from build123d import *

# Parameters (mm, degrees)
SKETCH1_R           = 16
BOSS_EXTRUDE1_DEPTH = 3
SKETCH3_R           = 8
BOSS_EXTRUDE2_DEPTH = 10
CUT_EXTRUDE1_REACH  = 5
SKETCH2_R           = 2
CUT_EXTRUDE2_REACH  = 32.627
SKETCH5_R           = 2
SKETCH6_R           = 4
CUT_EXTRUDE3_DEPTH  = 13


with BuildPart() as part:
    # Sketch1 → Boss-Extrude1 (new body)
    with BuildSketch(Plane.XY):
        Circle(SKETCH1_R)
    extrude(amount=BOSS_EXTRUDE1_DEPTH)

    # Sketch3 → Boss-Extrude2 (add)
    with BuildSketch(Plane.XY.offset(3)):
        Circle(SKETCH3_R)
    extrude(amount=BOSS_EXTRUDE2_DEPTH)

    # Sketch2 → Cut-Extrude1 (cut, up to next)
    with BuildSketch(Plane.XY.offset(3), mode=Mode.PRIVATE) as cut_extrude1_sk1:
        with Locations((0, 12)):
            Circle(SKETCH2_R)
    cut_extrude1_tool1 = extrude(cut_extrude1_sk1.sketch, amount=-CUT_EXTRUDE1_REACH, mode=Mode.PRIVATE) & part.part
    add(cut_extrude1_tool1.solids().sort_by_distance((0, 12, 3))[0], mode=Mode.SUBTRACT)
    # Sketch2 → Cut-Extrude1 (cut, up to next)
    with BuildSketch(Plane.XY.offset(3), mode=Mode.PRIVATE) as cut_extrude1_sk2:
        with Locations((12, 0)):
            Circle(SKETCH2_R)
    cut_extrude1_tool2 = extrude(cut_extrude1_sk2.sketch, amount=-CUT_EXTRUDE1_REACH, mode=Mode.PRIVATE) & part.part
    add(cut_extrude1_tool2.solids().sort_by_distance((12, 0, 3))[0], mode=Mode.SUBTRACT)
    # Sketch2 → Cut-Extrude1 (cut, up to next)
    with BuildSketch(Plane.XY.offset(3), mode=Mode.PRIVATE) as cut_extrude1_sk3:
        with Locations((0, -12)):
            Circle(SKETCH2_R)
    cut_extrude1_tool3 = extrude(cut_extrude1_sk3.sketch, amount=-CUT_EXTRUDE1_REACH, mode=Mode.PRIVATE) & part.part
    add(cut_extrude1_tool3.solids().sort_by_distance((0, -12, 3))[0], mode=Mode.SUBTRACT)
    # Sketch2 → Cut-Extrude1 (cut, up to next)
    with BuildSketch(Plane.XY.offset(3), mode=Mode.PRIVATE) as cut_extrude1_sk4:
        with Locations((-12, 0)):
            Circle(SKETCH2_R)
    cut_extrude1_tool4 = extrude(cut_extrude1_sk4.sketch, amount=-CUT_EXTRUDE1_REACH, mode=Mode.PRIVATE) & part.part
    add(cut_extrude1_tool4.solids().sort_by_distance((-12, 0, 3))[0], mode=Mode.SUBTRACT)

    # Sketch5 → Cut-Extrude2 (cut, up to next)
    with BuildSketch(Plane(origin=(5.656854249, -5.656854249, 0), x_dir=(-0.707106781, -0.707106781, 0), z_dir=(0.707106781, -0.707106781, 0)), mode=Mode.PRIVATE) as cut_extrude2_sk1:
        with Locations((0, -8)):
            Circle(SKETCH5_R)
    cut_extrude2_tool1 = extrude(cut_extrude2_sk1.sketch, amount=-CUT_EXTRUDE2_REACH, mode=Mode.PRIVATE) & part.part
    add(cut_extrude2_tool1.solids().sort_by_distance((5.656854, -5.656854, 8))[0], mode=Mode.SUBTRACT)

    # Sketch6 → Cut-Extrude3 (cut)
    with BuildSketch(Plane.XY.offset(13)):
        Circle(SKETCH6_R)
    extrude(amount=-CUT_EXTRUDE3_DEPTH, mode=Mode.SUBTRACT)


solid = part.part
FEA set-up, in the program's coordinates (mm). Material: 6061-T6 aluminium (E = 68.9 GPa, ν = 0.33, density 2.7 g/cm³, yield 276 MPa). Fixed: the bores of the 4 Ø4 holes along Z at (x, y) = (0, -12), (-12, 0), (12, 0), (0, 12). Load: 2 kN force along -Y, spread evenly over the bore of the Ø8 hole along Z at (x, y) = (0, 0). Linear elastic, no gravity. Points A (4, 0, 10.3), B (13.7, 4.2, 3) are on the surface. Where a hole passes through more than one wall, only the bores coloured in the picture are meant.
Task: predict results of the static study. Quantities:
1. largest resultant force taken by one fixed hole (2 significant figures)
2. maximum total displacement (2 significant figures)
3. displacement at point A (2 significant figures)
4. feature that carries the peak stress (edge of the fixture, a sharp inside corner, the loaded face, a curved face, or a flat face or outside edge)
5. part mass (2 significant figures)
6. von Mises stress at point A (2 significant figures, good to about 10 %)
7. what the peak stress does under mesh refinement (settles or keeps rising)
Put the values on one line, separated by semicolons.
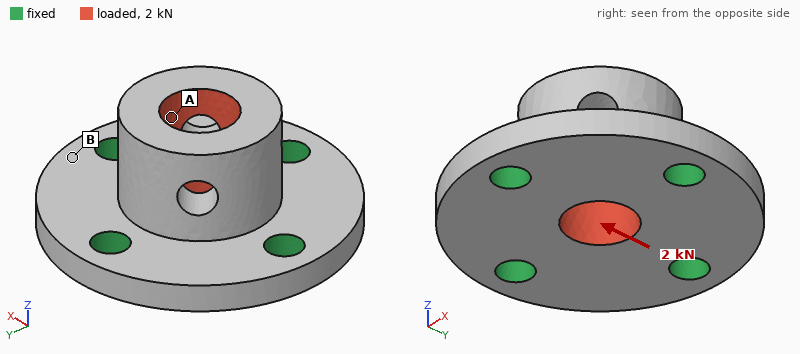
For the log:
800 N; 13 µm; 9.9 µm; edge of the fixture; 9.5 g; 19 MPa; keeps rising
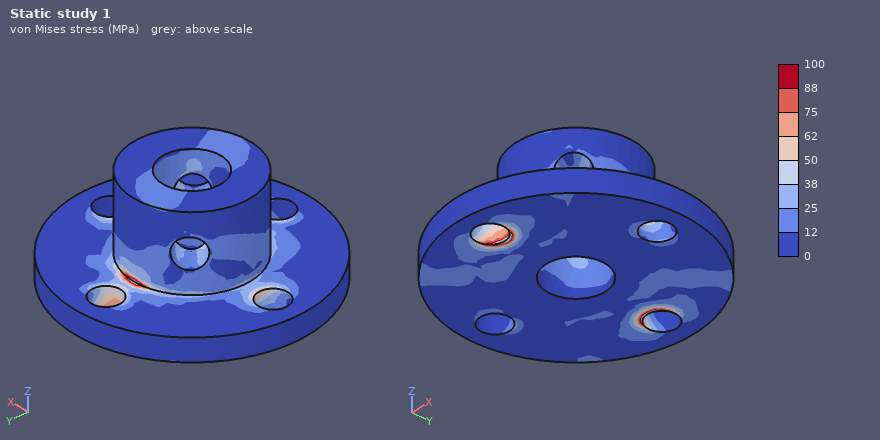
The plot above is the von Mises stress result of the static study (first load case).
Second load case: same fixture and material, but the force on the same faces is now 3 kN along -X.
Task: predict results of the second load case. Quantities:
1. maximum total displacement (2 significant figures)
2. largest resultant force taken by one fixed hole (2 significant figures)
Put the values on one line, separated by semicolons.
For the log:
20 µm; 1.2 kN
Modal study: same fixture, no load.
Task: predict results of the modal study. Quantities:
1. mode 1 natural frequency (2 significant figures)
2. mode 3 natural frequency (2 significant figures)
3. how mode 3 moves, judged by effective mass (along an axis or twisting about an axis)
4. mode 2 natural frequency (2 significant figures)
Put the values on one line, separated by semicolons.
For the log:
30 kHz; 38 kHz; along Z; 32 kHz
